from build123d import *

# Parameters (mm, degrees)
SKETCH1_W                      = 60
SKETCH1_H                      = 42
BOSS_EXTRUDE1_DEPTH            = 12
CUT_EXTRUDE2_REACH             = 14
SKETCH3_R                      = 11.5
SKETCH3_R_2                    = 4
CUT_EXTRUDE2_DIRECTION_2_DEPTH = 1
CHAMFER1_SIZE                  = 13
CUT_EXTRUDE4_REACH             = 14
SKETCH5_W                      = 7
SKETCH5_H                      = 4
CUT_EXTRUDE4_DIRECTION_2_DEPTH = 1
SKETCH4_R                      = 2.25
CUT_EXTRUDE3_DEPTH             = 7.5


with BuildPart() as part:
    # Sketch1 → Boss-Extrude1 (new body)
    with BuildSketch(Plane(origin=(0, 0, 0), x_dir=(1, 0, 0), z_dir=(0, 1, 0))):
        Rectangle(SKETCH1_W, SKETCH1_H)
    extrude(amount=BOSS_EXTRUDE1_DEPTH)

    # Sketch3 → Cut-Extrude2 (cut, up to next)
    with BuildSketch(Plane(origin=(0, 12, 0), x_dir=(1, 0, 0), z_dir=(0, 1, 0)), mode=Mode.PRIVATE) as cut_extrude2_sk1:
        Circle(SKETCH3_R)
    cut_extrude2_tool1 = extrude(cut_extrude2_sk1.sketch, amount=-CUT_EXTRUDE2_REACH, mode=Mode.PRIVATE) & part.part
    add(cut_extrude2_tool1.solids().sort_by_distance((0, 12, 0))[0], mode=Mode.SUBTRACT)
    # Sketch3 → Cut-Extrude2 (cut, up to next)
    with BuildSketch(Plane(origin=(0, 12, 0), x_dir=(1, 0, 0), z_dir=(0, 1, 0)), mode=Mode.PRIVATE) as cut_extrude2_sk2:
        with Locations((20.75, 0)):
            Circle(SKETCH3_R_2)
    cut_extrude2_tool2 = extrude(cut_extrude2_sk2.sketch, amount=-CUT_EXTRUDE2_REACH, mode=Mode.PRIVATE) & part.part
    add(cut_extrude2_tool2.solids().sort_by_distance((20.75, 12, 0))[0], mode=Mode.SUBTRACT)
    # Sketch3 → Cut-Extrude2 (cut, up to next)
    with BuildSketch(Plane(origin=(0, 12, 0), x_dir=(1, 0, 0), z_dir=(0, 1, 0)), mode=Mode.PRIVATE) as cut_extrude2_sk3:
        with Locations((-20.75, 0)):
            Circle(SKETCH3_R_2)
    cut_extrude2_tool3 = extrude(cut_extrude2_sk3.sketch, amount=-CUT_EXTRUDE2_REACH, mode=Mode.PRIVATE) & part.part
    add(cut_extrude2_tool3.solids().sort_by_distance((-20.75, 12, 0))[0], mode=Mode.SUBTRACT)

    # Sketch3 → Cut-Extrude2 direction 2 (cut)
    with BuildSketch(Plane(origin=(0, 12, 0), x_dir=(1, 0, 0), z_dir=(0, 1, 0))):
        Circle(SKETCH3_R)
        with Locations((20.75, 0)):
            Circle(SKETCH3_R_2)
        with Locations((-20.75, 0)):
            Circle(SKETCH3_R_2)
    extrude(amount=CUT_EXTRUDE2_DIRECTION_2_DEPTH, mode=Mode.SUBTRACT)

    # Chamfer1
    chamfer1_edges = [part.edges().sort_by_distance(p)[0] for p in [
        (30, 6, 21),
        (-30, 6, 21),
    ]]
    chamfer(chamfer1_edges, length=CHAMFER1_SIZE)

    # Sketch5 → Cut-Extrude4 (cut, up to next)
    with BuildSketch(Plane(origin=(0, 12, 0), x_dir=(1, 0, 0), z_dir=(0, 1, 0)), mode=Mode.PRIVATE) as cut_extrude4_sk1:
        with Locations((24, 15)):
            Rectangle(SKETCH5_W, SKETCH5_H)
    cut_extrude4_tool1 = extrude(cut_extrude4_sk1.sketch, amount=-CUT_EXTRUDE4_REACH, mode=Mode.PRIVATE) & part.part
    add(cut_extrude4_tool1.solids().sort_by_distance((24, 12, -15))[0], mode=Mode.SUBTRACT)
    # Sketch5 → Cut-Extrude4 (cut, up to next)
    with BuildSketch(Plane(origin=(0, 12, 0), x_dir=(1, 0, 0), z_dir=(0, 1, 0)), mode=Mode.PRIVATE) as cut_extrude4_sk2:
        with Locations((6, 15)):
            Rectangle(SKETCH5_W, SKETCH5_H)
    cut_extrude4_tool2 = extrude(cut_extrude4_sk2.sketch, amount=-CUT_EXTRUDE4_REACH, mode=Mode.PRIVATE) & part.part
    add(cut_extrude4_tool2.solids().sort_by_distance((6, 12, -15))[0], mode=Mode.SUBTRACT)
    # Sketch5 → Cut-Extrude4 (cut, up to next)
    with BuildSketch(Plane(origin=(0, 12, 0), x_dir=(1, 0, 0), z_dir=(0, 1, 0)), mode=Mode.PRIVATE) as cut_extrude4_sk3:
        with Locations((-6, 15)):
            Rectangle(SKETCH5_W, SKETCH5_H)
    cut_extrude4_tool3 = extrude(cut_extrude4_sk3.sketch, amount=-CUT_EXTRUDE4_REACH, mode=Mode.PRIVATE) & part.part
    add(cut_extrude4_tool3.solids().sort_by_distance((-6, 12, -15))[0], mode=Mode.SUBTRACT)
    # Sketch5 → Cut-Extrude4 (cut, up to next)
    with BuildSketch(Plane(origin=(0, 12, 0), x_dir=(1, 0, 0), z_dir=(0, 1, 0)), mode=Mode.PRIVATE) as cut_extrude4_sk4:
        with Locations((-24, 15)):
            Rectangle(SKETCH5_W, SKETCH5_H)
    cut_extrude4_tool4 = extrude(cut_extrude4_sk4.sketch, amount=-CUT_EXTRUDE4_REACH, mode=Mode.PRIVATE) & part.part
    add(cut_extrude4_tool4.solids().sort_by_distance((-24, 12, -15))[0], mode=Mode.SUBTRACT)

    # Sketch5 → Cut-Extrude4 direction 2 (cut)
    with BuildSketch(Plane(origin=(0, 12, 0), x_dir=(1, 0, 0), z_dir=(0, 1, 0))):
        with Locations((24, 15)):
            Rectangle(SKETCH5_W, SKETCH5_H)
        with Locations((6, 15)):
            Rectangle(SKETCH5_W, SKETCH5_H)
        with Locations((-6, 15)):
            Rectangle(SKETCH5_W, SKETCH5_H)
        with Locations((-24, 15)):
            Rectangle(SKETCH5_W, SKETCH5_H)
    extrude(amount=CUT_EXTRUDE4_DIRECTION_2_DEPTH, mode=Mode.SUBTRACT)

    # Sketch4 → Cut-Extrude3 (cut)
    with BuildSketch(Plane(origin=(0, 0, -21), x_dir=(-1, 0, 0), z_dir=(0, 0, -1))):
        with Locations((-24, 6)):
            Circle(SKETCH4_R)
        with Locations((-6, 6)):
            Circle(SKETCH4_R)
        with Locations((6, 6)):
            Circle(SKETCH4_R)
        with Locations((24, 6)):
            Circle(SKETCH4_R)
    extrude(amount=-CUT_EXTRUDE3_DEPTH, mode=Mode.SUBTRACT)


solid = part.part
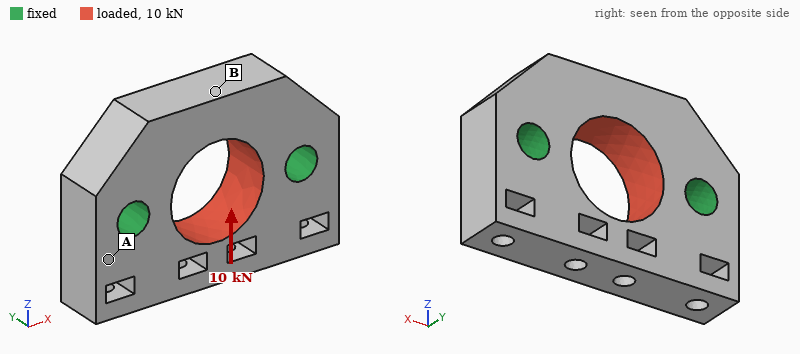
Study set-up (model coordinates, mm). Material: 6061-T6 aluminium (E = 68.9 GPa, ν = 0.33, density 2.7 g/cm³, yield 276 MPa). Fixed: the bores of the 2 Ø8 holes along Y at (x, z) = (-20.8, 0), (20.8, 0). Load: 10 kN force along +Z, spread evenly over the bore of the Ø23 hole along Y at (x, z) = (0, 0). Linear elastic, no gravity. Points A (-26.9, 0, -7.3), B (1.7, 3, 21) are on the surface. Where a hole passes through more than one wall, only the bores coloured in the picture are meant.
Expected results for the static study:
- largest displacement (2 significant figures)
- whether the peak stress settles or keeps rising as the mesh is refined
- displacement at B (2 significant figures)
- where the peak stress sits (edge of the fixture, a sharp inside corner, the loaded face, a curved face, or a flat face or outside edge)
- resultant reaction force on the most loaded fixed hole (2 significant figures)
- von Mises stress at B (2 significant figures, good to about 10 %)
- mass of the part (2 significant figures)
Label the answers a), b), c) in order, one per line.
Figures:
a) 18 µm
b) keeps rising
c) 8.6 µm
d) edge of the fixture
e) 5.0 kN
f) 29 MPa
g) 55 g
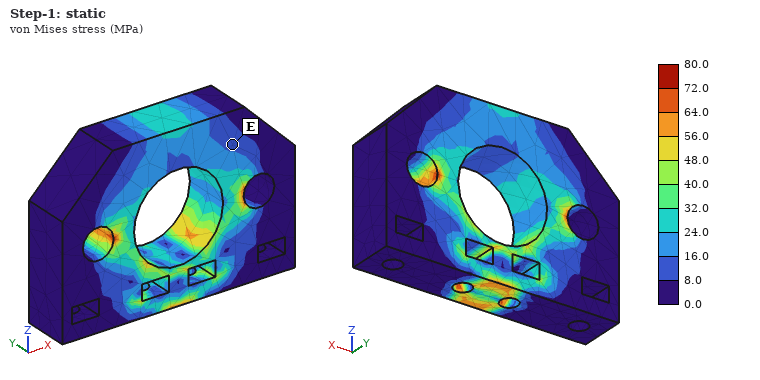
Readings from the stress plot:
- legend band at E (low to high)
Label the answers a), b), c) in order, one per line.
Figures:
a) 8.0 to 16.0 MPa
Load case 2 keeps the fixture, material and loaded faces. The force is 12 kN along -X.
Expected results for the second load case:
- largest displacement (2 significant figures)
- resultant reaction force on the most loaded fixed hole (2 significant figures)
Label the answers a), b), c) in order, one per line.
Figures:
a) 9.8 µm
b) 6.0 kN
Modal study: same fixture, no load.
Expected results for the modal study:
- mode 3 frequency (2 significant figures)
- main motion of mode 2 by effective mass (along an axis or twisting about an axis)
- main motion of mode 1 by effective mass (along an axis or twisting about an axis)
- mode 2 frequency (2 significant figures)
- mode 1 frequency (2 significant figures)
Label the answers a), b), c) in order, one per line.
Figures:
a) 23 kHz
b) along Y
c) twisting about X
d) 17 kHz
e) 16 kHz
